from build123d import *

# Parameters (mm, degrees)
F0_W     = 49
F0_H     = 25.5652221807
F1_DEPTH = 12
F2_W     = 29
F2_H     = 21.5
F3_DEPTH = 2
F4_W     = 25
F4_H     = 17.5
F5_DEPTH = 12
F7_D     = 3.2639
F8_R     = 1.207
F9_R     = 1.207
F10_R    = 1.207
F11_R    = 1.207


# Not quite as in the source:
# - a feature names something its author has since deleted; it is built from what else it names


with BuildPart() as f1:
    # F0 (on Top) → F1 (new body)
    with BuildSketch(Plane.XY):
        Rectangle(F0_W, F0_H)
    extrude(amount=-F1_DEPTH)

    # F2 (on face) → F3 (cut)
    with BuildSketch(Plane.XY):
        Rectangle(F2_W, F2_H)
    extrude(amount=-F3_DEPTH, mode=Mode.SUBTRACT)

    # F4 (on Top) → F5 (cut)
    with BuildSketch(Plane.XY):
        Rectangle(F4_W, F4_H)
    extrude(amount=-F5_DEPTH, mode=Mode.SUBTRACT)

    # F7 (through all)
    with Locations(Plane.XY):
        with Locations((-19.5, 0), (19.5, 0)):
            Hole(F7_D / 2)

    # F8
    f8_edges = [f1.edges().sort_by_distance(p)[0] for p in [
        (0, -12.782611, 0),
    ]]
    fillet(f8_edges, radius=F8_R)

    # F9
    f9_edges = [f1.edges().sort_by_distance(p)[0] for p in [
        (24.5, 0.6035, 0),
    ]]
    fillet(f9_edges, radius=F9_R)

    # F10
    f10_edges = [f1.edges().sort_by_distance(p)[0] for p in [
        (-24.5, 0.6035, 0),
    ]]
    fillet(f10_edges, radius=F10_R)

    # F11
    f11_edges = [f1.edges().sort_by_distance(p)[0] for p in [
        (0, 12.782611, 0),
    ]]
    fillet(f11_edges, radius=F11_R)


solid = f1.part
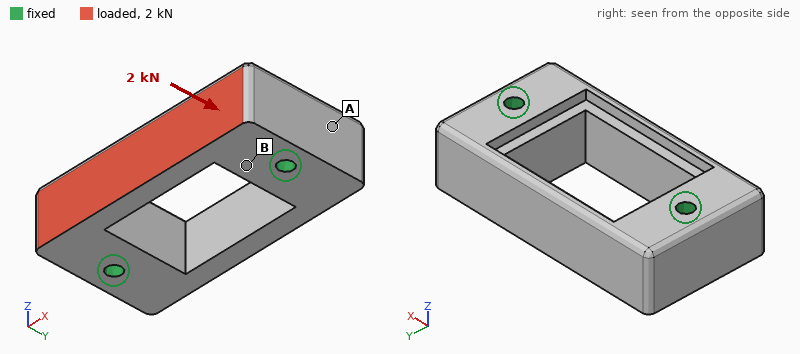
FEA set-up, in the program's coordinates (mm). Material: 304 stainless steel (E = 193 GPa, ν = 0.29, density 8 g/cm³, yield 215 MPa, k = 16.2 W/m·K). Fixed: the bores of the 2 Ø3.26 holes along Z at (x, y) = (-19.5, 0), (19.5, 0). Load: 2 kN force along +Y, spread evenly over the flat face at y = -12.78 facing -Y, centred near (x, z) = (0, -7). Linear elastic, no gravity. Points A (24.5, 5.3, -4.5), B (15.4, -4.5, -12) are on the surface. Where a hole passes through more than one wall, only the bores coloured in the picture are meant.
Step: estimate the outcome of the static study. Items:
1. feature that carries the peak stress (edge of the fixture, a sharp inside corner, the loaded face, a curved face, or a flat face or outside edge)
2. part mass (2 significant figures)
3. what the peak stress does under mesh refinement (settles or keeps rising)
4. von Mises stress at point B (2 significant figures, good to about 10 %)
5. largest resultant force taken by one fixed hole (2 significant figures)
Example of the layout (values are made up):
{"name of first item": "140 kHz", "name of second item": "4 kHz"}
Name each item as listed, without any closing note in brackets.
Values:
{"feature that carries the peak stress": "a sharp inside corner", "part mass": "73 g", "what the peak stress does under mesh refinement": "keeps rising", "von Mises stress at point B": "18 MPa", "largest resultant force taken by one fixed hole": "1.1 kN"}
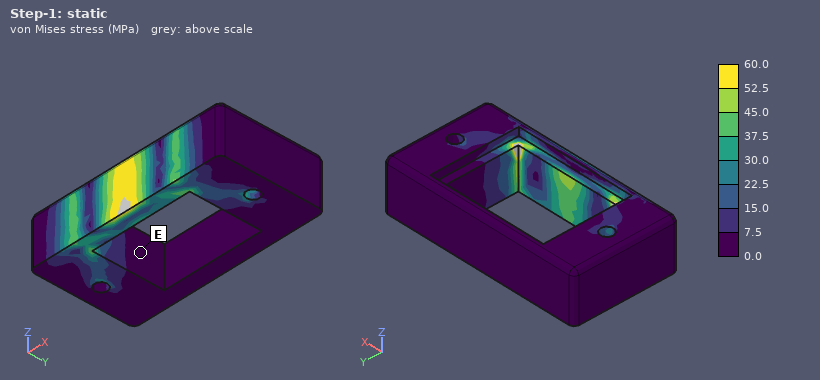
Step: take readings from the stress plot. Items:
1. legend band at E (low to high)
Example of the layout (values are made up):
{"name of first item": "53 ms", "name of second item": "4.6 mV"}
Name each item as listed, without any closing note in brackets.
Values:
{"legend band at E": "0.0 to 7.5 MPa"}
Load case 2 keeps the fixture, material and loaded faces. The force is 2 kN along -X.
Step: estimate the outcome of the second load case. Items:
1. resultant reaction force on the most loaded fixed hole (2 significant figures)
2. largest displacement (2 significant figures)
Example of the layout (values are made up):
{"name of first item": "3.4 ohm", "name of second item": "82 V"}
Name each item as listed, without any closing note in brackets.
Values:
{"resultant reaction force on the most loaded fixed hole": "1.0 kN", "largest displacement": "5.8 µm"}
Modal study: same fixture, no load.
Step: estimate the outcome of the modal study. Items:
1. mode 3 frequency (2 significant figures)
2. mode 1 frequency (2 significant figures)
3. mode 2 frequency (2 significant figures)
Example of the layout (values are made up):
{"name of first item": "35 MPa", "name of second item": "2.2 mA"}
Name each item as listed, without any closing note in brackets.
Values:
{"mode 3 frequency": "20 kHz", "mode 1 frequency": "17 kHz", "mode 2 frequency": "20 kHz"}
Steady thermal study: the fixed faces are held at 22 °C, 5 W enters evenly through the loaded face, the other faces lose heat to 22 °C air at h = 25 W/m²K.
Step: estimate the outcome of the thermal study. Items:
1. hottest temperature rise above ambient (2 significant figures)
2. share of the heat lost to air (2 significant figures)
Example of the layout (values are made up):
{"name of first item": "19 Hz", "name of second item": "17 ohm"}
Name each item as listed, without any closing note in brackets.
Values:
{"hottest temperature rise above ambient": "27 K", "share of the heat lost to air": "10 %"}
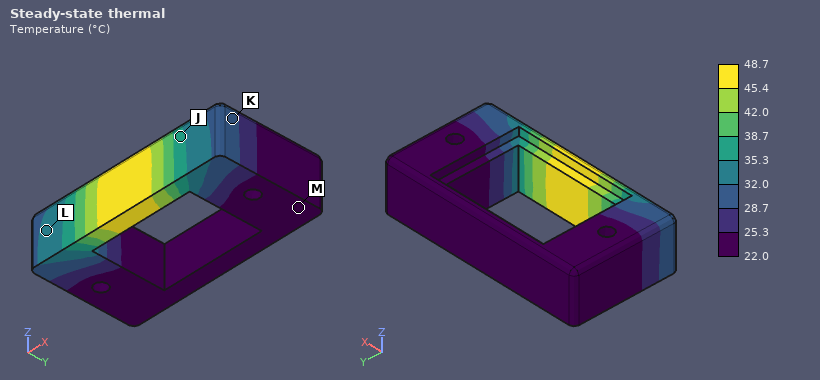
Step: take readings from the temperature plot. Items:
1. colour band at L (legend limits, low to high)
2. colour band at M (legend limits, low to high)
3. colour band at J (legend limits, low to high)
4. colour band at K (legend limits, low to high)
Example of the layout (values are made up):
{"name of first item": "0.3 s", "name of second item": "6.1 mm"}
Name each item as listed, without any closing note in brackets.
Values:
{"colour band at L": "32.0 to 35.3 °C", "colour band at M": "22.0 to 25.3 °C", "colour band at J": "35.3 to 38.7 °C", "colour band at K": "28.7 to 32.0 °C"}
